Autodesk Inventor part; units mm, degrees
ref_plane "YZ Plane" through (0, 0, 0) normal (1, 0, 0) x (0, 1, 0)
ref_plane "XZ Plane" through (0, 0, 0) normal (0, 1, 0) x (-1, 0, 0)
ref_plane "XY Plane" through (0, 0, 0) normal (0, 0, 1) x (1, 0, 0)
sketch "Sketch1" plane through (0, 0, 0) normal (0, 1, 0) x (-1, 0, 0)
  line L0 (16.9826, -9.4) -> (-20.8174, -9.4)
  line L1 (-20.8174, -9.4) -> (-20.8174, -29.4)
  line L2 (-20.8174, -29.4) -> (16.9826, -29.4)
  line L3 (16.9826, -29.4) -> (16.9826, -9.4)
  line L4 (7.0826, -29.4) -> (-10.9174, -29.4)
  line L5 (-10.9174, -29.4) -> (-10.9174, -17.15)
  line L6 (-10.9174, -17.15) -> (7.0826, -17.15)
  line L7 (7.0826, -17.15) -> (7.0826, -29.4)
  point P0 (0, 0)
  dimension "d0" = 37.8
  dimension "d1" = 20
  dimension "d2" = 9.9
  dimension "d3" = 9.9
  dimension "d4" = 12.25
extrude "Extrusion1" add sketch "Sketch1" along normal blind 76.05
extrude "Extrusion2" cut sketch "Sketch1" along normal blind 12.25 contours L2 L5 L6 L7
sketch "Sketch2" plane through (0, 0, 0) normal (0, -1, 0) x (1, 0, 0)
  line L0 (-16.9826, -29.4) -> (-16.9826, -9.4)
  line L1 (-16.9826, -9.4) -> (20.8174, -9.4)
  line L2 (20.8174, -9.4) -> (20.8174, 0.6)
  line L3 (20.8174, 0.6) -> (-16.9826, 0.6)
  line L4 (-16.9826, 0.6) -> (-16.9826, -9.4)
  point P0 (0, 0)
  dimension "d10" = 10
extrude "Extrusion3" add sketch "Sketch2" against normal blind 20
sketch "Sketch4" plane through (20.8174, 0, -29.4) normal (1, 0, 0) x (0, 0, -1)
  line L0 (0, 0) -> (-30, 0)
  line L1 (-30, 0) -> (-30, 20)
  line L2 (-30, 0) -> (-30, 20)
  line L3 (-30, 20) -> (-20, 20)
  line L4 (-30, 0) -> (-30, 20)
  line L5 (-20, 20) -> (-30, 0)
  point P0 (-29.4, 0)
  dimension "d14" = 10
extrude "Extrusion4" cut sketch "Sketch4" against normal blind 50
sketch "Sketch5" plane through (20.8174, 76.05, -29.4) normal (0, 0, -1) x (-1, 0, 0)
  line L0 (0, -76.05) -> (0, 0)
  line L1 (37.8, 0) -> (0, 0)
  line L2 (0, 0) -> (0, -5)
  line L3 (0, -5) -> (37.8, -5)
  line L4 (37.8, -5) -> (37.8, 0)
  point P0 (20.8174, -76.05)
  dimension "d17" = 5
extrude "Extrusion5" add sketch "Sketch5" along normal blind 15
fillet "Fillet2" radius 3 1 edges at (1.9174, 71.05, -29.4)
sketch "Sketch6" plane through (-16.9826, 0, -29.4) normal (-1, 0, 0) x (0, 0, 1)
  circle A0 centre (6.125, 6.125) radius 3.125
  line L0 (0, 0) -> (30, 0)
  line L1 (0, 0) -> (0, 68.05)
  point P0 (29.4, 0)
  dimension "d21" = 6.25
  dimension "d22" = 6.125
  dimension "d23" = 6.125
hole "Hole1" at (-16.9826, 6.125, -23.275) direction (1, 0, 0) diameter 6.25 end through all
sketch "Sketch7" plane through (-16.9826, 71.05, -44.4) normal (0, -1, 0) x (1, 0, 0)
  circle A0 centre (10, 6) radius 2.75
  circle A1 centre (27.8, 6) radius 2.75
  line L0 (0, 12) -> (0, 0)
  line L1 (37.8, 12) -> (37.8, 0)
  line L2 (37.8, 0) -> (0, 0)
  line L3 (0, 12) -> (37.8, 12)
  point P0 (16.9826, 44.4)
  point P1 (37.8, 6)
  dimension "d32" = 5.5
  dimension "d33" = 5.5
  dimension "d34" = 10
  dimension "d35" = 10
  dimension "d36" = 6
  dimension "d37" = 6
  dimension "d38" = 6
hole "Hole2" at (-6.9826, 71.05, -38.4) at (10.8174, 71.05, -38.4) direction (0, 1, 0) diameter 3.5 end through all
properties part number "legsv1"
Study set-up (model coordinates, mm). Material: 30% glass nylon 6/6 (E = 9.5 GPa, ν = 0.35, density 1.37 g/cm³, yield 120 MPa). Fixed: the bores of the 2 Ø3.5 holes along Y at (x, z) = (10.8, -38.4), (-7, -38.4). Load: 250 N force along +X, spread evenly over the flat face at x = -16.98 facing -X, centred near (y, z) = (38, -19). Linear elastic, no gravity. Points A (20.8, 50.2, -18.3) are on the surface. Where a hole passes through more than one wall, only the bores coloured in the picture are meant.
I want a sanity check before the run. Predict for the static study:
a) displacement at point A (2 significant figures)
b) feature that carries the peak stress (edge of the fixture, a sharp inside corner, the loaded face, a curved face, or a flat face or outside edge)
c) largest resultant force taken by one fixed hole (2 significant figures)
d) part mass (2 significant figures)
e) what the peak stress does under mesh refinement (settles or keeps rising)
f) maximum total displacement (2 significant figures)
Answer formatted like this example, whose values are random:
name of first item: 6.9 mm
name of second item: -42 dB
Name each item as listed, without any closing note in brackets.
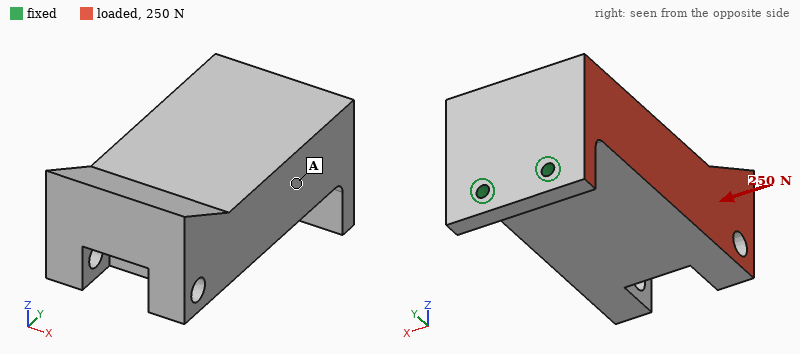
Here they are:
displacement at point A: 0.14 mm
feature that carries the peak stress: edge of the fixture
largest resultant force taken by one fixed hole: 470 N
part mass: 83 g
what the peak stress does under mesh refinement: keeps rising
maximum total displacement: 0.35 mm
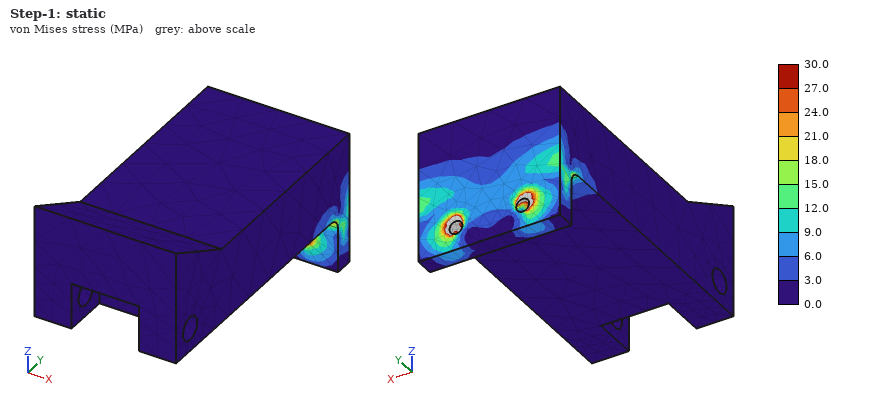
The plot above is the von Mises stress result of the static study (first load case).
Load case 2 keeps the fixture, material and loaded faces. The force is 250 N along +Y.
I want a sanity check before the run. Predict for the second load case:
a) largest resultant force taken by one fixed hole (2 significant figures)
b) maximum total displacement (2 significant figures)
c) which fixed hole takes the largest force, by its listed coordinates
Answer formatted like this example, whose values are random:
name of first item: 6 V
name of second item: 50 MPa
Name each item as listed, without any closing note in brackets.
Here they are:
largest resultant force taken by one fixed hole: 330 N
maximum total displacement: 0.88 mm
which fixed hole takes the largest force, by its listed coordinates: (-7, -38.4)
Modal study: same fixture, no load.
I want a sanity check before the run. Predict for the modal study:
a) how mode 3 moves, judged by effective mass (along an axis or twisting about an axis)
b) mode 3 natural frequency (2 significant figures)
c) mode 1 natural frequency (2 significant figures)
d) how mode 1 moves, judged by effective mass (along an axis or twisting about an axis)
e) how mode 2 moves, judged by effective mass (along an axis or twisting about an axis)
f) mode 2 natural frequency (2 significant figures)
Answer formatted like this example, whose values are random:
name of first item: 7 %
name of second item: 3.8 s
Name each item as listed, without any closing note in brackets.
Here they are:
how mode 3 moves, judged by effective mass: along Y
mode 3 natural frequency: 2300 Hz
mode 1 natural frequency: 230 Hz
how mode 1 moves, judged by effective mass: along Z
how mode 2 moves, judged by effective mass: along X
mode 2 natural frequency: 570 Hz
